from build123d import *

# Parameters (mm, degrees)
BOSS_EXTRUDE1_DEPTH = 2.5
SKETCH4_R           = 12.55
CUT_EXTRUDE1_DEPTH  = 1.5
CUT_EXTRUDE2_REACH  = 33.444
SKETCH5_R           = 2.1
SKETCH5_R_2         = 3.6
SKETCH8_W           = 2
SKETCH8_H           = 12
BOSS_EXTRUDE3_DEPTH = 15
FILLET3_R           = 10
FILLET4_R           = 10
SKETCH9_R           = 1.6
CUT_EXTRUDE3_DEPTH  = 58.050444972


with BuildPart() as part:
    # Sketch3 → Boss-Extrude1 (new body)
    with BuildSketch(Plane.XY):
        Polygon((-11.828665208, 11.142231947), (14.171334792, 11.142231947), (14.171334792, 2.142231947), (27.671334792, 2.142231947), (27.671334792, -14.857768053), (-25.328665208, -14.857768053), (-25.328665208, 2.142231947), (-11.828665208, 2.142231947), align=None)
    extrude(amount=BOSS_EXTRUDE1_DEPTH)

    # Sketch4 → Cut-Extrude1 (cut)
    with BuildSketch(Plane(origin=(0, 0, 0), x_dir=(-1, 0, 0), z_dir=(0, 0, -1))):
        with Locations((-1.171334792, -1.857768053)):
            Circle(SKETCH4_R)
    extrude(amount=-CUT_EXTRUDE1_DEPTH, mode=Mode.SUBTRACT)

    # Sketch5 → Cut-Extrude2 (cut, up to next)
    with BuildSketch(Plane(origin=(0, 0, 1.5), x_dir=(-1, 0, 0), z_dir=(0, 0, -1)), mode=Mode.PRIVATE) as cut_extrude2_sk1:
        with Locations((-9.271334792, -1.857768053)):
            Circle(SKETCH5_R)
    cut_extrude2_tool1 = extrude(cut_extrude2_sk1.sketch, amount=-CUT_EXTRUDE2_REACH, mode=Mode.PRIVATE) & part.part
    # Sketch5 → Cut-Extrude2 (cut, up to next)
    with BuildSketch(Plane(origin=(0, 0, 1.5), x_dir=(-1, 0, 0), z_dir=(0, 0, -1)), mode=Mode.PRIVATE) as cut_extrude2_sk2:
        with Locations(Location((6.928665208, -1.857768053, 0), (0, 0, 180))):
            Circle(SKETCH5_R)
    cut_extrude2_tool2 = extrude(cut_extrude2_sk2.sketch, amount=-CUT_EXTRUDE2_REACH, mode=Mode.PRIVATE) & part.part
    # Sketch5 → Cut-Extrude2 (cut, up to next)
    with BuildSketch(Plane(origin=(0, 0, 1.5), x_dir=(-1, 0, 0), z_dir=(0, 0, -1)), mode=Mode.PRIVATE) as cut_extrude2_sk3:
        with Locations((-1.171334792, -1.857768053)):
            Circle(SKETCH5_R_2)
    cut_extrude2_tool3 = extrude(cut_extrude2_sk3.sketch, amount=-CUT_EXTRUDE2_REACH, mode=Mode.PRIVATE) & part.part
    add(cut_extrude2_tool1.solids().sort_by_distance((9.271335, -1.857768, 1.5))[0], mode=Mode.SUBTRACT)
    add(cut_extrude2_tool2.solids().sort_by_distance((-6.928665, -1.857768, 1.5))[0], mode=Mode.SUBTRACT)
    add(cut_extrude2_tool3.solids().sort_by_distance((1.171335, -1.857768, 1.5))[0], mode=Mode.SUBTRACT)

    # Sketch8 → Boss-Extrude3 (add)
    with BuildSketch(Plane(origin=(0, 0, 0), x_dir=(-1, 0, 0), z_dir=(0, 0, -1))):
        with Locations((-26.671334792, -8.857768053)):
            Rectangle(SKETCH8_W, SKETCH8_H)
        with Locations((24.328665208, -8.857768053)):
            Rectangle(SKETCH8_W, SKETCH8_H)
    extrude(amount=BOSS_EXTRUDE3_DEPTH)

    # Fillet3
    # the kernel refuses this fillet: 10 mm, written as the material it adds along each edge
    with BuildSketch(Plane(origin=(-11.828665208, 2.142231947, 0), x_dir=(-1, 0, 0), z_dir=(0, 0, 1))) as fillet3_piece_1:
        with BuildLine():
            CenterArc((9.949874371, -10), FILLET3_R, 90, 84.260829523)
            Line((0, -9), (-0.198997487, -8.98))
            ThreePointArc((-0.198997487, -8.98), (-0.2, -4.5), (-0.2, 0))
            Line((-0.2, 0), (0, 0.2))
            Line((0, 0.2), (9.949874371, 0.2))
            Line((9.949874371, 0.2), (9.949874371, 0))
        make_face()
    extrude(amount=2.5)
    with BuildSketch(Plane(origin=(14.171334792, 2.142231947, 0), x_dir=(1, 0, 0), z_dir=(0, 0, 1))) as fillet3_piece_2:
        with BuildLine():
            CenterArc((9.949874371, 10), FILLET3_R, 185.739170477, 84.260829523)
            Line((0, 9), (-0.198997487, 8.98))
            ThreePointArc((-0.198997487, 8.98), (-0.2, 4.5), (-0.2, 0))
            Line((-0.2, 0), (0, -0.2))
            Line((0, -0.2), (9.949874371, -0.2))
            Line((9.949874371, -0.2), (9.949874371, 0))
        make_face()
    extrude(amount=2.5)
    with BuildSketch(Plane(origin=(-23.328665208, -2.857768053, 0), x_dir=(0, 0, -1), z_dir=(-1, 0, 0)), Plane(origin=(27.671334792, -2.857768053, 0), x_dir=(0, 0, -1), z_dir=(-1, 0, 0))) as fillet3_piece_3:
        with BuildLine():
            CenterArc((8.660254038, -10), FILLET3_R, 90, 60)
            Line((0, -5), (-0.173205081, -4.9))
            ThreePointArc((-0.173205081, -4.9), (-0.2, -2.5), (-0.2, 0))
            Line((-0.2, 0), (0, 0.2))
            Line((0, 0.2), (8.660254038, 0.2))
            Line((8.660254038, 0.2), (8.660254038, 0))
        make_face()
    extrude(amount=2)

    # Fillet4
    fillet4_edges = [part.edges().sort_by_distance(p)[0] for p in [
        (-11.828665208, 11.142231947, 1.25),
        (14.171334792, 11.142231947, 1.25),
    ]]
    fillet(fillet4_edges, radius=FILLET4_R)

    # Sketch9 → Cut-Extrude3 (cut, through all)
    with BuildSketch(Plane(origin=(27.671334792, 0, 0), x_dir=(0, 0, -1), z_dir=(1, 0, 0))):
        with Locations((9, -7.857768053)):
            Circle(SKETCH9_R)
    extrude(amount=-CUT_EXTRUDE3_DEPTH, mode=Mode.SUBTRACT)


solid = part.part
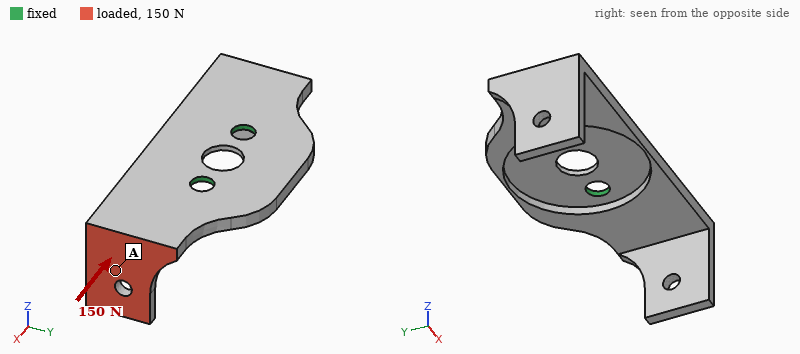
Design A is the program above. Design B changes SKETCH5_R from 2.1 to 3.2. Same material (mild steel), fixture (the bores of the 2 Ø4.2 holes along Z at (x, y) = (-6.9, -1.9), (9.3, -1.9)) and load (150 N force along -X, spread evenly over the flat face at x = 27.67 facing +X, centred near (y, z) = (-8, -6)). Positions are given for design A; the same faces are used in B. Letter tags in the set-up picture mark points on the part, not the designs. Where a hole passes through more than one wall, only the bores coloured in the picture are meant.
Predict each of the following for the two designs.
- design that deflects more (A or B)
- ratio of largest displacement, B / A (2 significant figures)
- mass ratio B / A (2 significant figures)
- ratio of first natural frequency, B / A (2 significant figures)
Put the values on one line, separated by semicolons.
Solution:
A; 0.84; 0.99; 1.2
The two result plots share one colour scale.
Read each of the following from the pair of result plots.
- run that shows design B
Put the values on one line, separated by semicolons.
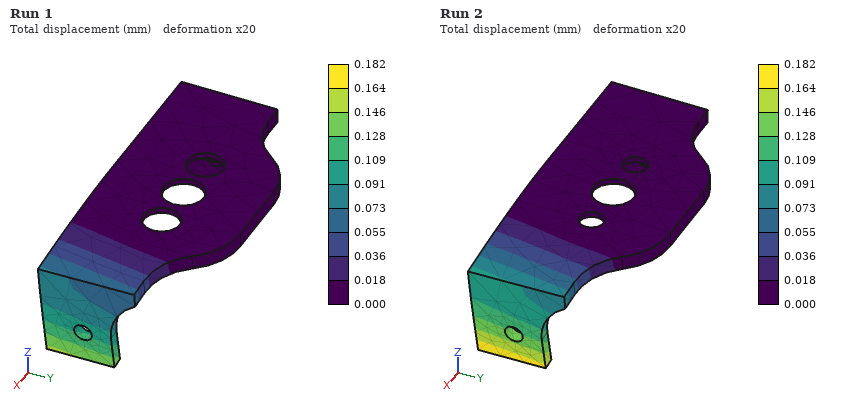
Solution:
Run 1
